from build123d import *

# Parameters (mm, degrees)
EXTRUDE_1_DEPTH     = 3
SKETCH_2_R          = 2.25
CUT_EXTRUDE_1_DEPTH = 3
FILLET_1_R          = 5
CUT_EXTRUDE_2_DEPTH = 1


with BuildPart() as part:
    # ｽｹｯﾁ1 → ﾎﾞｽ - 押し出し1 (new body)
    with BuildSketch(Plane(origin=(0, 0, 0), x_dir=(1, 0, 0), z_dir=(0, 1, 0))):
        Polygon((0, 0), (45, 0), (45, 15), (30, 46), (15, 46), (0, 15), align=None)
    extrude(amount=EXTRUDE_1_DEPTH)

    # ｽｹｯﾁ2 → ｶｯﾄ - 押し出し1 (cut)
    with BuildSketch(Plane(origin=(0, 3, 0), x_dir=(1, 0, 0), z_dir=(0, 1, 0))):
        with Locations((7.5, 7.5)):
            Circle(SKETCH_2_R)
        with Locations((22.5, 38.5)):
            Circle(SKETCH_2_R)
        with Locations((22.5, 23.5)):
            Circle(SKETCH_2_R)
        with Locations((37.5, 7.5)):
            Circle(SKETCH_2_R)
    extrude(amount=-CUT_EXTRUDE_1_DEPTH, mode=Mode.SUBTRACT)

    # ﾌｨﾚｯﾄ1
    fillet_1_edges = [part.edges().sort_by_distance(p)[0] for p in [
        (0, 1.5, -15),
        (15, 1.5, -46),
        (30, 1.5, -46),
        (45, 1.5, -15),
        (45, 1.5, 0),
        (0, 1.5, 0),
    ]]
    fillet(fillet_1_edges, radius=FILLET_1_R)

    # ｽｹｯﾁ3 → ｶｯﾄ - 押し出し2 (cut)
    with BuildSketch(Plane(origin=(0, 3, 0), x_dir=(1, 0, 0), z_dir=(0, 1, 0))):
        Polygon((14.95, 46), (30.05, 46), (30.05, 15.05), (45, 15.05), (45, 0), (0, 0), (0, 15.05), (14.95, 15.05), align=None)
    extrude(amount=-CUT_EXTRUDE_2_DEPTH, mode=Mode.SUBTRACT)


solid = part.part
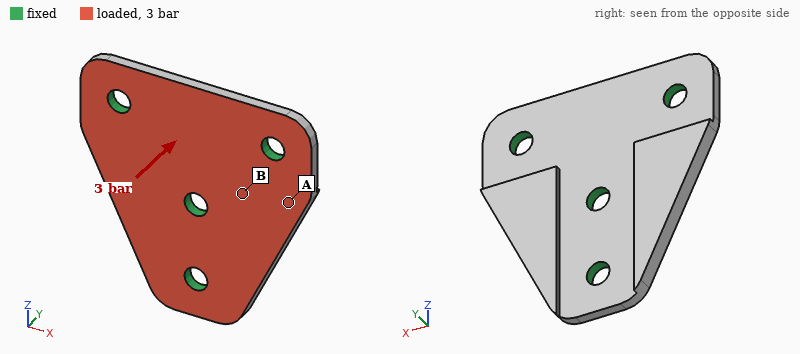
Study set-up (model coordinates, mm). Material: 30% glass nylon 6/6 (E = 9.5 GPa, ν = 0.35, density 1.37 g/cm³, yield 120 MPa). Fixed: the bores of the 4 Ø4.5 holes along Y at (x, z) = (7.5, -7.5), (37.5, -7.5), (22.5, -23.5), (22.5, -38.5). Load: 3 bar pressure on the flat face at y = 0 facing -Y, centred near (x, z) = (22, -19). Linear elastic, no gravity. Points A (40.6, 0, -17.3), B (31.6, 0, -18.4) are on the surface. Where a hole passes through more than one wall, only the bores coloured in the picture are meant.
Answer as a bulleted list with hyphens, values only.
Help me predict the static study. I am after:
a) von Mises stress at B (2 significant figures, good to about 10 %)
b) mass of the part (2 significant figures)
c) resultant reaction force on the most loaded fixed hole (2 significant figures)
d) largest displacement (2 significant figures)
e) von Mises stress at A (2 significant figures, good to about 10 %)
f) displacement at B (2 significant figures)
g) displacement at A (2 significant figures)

- 10 MPa
- 4.8 g
- 120 N
- 99 µm
- 4.5 MPa
- 29 µm
- 55 µm
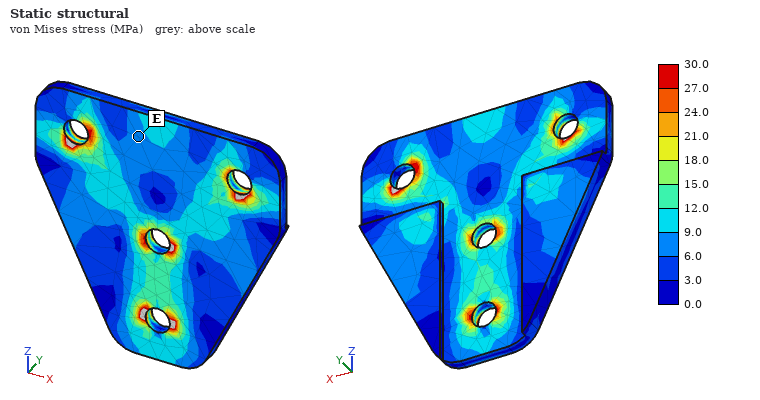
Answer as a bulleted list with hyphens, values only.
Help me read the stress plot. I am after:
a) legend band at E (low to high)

- 6.0 to 9.0 MPa
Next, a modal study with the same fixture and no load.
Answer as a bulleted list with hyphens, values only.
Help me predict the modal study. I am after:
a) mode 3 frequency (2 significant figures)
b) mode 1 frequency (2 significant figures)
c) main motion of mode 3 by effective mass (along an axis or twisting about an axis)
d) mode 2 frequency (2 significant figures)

- 7500 Hz
- 5500 Hz
- along Y
- 5600 Hz
